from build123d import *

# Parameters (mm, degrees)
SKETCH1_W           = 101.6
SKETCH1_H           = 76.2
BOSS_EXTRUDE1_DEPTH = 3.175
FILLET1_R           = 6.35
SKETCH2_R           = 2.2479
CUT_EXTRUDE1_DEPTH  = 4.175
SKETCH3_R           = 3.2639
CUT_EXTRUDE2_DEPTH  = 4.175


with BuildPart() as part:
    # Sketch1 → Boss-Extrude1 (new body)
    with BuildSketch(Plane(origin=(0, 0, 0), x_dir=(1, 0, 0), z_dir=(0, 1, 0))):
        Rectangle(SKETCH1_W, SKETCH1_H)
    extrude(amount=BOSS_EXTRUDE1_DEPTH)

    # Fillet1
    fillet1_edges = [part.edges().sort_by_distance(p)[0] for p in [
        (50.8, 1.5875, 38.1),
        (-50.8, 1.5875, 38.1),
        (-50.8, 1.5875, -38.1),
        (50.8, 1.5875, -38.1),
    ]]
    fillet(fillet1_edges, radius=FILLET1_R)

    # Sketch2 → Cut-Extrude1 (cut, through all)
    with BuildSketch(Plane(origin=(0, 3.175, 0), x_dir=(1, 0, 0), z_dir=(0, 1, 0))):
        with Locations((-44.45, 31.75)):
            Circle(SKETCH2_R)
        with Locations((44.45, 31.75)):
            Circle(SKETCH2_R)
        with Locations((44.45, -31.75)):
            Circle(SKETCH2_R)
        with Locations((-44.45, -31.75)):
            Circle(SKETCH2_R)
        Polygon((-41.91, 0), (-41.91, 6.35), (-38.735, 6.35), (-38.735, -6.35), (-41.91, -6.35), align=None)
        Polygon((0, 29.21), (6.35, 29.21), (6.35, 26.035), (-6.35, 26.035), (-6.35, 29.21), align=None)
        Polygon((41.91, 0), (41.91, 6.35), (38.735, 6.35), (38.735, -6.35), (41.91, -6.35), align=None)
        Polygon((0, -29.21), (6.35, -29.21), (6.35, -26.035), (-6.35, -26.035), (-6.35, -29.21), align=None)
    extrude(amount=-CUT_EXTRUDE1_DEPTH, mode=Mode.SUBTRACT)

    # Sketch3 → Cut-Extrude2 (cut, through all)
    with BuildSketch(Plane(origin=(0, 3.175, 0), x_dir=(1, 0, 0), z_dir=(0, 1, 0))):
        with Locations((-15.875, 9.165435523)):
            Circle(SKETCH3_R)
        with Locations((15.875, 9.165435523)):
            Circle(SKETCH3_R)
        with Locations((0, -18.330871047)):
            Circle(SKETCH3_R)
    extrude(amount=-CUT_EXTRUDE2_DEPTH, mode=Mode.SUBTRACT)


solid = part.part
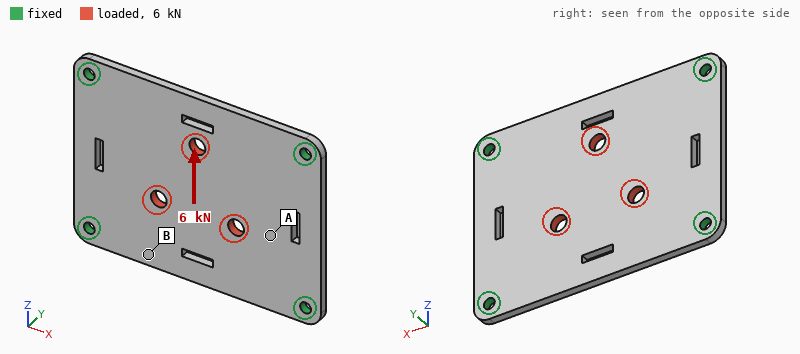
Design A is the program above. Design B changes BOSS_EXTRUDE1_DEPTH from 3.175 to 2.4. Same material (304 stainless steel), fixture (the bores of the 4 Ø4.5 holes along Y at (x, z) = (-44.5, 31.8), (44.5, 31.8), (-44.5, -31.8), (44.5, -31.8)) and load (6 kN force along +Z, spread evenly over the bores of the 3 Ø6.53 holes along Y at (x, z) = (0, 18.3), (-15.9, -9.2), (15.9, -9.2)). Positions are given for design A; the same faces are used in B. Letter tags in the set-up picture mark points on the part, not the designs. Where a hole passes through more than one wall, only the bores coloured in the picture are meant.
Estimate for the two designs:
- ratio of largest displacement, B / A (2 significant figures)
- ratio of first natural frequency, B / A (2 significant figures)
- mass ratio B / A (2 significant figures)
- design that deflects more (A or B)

1.3
0.77
0.76
B
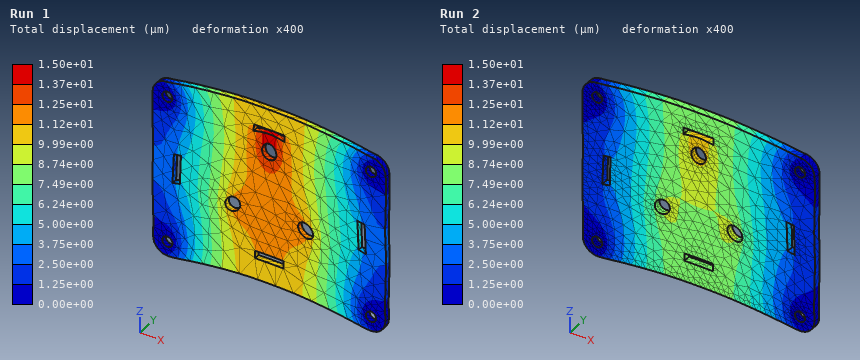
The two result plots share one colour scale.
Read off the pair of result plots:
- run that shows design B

Run 1
